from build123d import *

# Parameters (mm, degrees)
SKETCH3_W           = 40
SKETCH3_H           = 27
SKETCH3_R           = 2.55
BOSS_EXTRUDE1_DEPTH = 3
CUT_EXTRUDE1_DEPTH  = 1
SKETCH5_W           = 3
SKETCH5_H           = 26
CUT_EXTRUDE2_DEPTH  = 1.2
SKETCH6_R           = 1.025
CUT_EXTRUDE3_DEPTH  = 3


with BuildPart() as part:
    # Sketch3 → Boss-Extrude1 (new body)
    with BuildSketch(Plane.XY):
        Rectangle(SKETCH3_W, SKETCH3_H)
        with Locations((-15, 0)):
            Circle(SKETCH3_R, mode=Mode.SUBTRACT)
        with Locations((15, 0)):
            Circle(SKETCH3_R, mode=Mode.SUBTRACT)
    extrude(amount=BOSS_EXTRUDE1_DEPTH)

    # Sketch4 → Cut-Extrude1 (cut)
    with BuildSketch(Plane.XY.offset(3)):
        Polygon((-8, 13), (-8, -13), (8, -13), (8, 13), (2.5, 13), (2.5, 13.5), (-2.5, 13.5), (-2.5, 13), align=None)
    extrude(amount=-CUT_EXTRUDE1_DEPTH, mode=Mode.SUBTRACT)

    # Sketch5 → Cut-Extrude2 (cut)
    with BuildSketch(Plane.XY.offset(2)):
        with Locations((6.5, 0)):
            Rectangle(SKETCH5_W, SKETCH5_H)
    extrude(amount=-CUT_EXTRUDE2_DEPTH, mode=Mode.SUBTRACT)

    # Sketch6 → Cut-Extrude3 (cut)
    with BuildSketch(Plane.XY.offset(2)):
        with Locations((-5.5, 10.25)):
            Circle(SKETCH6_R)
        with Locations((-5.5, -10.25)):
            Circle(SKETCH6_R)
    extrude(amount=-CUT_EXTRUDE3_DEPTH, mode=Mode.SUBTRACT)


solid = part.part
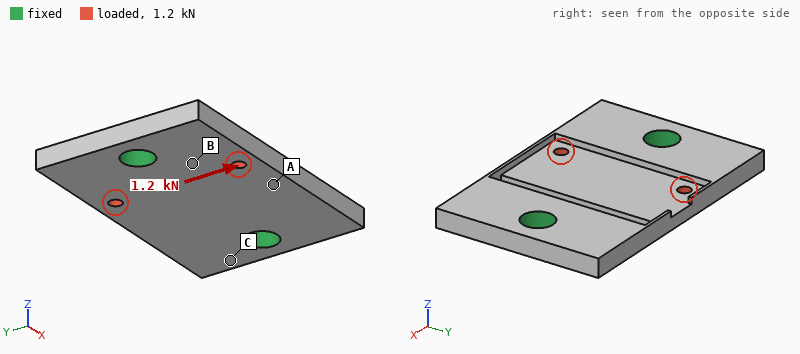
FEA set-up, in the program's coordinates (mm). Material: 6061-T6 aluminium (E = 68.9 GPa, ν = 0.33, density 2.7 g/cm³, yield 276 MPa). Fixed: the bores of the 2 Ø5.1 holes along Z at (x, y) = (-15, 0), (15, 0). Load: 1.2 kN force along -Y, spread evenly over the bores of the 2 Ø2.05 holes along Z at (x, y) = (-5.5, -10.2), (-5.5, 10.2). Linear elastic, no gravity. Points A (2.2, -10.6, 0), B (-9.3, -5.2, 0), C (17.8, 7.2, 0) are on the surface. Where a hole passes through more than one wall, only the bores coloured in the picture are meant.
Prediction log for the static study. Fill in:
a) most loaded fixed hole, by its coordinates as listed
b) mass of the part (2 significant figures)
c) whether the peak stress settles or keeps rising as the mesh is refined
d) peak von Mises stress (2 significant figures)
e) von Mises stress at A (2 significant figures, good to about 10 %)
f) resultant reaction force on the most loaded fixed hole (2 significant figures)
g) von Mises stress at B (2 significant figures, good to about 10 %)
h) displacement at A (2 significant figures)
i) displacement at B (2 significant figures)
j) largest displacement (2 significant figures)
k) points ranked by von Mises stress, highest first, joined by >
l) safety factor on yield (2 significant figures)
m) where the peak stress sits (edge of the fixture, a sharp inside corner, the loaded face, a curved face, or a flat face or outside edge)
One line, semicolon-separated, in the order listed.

(-15, 0); 7.0 g; settles; 98 MPa; 16 MPa; 850 N; 31 MPa; 7.3 µm; 4.4 µm; 11 µm; B > A > C; 2.8; the loaded face
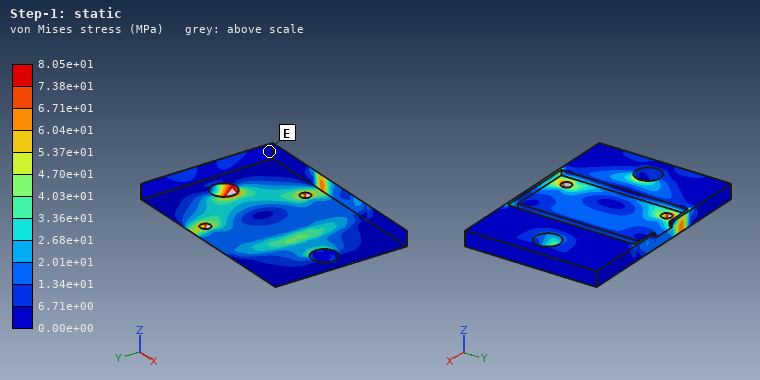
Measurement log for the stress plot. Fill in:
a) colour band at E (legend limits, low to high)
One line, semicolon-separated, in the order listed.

0.00e+00 to 6.71e+00 MPa
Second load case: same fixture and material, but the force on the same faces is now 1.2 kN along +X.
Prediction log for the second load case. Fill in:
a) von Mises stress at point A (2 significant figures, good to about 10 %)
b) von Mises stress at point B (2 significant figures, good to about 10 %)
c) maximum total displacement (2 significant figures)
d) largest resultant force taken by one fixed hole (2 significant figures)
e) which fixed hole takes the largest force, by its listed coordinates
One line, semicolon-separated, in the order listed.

17 MPa; 23 MPa; 8.2 µm; 830 N; (-15, 0)
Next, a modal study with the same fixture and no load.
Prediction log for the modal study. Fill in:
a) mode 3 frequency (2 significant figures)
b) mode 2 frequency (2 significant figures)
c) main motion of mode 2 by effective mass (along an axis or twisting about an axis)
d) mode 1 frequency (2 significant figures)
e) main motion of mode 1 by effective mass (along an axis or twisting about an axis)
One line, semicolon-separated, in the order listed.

18 kHz; 13 kHz; along Z; 12 kHz; twisting about X
